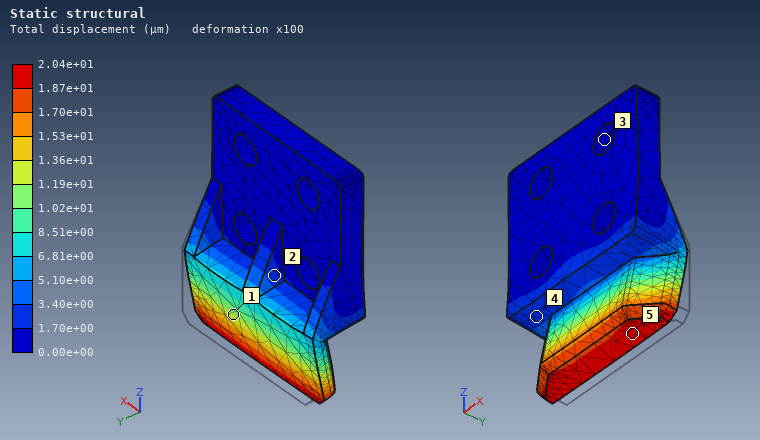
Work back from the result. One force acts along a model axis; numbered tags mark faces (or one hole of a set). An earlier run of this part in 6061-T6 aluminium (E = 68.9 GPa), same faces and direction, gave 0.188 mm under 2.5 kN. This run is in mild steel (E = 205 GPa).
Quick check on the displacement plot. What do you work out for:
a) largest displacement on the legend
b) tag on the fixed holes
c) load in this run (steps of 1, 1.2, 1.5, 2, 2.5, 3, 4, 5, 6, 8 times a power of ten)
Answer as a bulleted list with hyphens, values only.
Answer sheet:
- 2.04e+01 µm
- 3
- 800 N
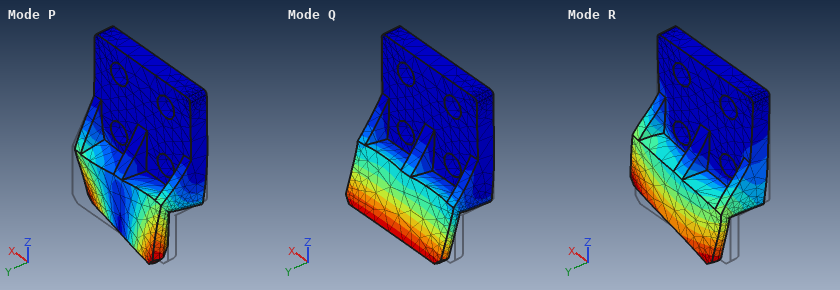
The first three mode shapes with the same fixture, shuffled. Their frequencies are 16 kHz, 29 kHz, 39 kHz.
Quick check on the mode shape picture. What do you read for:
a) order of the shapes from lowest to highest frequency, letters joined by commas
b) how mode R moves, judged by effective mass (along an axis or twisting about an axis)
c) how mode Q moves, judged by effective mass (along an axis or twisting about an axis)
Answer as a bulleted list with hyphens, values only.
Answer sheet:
- Q, P, R
- along X
- along Y
